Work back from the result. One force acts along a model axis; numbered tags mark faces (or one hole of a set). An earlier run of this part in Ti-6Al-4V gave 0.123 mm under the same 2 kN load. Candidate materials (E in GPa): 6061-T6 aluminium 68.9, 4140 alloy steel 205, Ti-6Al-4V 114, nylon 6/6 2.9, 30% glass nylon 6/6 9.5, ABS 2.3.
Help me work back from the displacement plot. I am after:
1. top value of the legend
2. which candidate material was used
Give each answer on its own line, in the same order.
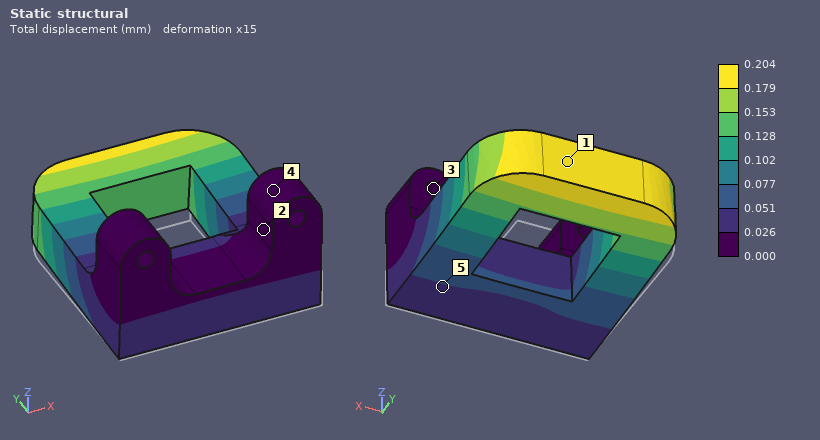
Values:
0.204 mm
6061-T6 aluminium
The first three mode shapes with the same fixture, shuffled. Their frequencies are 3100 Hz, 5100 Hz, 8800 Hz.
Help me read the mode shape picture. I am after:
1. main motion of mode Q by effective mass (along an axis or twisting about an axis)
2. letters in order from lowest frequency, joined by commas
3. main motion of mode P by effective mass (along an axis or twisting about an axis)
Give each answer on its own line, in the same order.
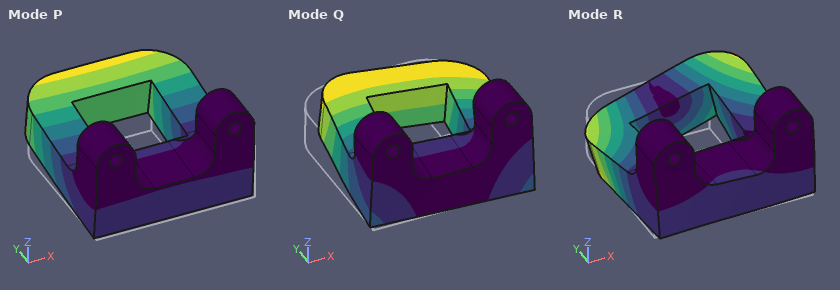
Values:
along X
P, Q, R
along Z
